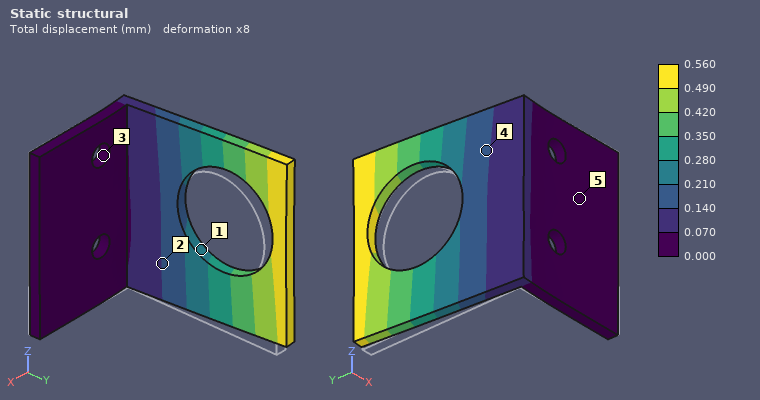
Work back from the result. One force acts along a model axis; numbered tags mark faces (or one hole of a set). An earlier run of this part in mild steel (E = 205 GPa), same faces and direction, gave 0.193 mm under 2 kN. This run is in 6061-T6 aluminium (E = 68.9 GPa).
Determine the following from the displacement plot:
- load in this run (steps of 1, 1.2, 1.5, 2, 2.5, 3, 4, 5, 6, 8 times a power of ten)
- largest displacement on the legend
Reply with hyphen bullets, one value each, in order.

- 2 kN
- 0.560 mm
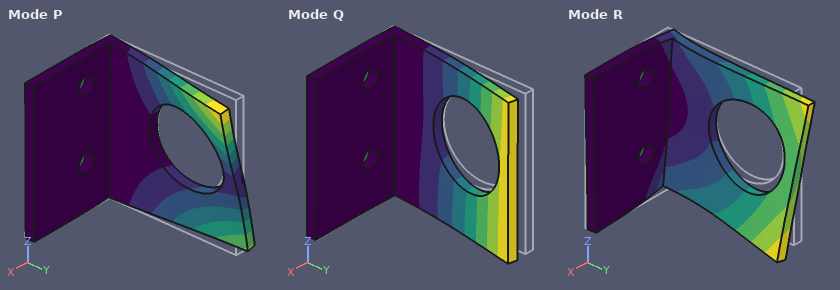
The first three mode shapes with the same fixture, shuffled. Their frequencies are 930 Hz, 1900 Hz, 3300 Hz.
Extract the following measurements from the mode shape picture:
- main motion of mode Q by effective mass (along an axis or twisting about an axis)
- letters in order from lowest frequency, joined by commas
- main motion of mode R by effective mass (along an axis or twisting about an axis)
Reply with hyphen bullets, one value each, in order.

- along X
- Q, P, R
- along Z
